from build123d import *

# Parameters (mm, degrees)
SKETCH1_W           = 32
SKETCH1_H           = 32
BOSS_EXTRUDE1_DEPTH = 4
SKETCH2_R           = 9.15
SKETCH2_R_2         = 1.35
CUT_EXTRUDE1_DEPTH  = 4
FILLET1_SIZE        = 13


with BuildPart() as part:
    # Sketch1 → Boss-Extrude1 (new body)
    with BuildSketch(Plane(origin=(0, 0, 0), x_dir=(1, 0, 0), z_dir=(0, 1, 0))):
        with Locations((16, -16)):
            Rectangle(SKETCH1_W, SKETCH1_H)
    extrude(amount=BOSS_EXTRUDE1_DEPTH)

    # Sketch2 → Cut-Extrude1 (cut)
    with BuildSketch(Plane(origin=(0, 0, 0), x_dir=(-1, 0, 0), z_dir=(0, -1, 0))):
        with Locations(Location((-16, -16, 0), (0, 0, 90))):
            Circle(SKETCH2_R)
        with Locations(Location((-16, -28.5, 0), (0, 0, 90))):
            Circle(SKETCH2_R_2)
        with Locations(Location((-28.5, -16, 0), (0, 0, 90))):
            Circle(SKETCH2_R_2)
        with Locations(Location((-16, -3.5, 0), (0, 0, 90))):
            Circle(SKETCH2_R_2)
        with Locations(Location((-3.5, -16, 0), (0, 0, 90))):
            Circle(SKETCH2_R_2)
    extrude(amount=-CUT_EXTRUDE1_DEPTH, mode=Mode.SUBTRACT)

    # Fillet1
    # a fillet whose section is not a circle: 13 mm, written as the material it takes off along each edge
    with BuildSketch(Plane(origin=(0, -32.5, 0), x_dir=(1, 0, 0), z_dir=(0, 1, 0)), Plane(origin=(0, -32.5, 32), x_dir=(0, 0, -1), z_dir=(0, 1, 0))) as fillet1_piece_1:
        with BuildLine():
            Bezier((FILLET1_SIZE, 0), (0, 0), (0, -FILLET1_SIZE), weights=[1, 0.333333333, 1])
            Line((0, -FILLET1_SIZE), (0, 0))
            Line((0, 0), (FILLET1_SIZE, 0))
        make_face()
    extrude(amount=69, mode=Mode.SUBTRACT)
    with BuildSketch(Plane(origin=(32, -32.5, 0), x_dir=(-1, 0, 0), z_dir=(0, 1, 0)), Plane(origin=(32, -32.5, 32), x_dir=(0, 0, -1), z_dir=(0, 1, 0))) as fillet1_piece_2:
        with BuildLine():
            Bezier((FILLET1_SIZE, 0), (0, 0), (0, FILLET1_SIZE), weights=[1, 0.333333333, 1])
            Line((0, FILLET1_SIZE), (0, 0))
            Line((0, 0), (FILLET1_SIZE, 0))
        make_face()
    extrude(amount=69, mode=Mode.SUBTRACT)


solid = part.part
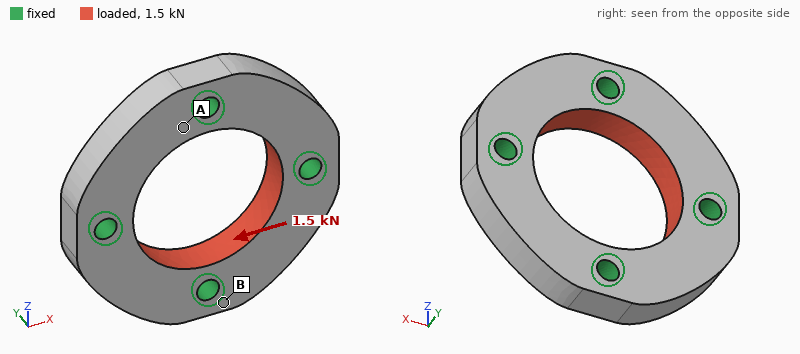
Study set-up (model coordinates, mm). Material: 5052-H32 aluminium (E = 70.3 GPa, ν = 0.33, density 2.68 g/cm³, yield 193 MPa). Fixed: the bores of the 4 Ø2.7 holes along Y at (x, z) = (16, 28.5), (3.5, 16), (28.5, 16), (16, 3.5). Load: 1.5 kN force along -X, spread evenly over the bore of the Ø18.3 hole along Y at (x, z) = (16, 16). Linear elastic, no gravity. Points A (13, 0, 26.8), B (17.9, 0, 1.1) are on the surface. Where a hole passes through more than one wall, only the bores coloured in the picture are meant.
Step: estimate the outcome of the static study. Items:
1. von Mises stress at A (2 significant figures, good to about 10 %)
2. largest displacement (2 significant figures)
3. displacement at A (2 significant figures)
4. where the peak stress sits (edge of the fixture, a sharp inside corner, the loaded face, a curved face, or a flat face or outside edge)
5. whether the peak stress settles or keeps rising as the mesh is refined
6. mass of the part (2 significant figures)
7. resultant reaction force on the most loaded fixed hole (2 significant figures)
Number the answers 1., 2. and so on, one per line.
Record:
1. 11 MPa
2. 1.7 µm
3. 0.67 µm
4. edge of the fixture
5. keeps rising
6. 5.6 g
7. 430 N
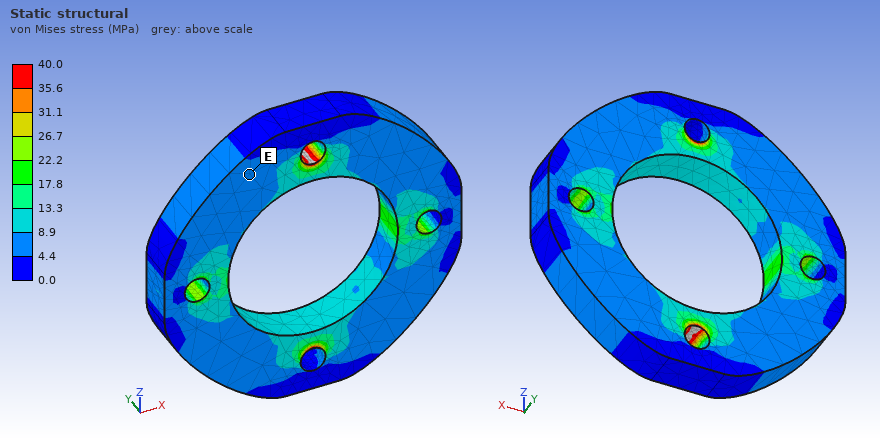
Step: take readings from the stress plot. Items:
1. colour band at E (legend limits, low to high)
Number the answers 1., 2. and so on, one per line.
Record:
1. 4.4 to 8.9 MPa
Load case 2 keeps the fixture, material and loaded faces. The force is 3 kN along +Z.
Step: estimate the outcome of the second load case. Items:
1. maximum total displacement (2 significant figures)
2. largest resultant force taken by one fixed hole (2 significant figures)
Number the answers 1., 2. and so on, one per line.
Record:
1. 3.4 µm
2. 860 N
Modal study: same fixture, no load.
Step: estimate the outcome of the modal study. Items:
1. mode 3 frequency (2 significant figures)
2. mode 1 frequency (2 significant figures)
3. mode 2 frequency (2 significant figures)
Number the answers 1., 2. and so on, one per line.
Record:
1. 43 kHz
2. 42 kHz
3. 43 kHz
